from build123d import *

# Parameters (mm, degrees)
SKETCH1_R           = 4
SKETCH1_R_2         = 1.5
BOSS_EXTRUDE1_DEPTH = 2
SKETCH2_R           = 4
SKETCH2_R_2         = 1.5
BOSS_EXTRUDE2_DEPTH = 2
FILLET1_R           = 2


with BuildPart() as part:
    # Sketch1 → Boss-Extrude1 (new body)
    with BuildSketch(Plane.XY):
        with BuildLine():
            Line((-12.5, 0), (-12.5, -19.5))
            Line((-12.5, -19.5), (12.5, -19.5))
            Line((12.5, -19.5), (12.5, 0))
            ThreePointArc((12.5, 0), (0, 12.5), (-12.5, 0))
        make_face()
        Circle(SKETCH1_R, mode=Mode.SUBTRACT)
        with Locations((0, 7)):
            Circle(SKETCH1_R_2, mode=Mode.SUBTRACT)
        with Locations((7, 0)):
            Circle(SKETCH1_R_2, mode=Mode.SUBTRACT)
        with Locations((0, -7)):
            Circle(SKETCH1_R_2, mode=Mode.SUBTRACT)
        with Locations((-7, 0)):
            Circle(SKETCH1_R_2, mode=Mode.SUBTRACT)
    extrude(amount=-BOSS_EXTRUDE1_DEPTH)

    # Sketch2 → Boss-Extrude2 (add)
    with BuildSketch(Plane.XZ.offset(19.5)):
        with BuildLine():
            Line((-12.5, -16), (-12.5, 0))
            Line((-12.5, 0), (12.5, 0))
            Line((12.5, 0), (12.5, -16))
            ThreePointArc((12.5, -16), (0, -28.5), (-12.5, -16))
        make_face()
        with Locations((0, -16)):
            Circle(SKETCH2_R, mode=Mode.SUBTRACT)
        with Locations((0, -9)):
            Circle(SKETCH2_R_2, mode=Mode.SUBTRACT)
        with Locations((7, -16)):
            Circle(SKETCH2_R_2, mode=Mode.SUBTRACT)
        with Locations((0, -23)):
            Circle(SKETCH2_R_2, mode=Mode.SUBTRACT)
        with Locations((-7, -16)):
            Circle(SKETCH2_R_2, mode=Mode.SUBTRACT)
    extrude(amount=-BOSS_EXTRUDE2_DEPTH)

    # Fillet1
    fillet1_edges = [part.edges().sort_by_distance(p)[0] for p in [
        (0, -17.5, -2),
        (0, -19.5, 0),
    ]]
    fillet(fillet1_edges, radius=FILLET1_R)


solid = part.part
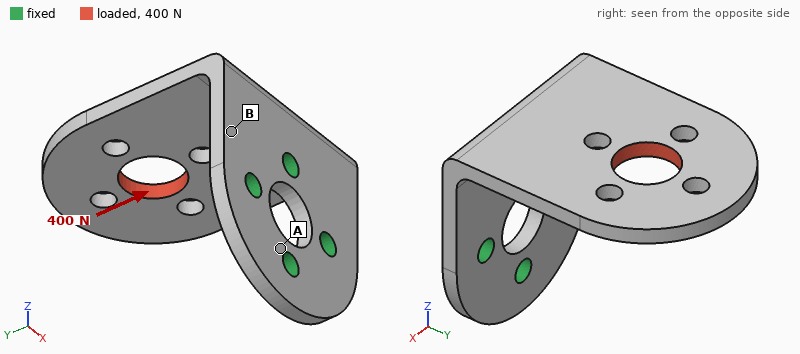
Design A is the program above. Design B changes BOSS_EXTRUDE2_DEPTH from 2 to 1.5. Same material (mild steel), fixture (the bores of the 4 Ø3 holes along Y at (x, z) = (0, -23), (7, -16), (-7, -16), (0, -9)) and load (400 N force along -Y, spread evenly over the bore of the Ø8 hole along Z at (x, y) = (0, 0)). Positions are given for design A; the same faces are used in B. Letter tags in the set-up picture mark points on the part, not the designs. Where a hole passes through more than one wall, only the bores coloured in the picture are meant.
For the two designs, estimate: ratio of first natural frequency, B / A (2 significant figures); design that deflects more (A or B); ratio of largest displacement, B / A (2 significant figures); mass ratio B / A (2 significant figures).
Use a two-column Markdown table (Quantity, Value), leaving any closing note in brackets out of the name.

| Quantity | Value |
|---|---|
| ratio of first natural frequency, B / A | 0.76 |
| design that deflects more | B |
| ratio of largest displacement, B / A | 2.2 |
| mass ratio B / A | 0.89 |
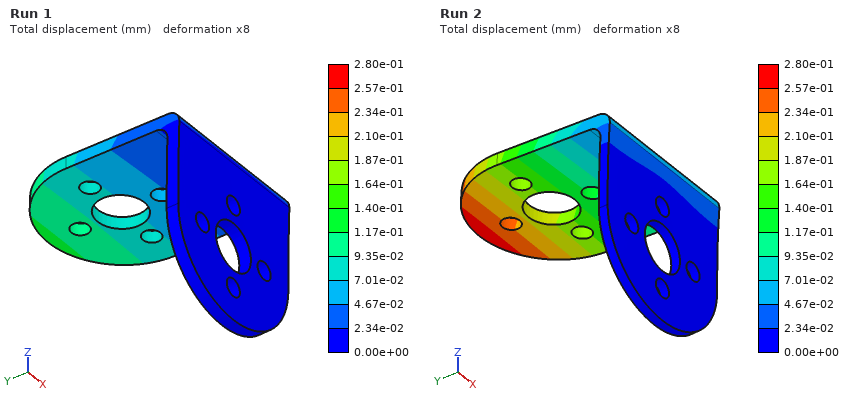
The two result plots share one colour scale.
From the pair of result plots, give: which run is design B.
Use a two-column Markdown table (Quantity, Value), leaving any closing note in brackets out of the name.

| Quantity | Value |
|---|---|
| which run is design B | Run 2 |
